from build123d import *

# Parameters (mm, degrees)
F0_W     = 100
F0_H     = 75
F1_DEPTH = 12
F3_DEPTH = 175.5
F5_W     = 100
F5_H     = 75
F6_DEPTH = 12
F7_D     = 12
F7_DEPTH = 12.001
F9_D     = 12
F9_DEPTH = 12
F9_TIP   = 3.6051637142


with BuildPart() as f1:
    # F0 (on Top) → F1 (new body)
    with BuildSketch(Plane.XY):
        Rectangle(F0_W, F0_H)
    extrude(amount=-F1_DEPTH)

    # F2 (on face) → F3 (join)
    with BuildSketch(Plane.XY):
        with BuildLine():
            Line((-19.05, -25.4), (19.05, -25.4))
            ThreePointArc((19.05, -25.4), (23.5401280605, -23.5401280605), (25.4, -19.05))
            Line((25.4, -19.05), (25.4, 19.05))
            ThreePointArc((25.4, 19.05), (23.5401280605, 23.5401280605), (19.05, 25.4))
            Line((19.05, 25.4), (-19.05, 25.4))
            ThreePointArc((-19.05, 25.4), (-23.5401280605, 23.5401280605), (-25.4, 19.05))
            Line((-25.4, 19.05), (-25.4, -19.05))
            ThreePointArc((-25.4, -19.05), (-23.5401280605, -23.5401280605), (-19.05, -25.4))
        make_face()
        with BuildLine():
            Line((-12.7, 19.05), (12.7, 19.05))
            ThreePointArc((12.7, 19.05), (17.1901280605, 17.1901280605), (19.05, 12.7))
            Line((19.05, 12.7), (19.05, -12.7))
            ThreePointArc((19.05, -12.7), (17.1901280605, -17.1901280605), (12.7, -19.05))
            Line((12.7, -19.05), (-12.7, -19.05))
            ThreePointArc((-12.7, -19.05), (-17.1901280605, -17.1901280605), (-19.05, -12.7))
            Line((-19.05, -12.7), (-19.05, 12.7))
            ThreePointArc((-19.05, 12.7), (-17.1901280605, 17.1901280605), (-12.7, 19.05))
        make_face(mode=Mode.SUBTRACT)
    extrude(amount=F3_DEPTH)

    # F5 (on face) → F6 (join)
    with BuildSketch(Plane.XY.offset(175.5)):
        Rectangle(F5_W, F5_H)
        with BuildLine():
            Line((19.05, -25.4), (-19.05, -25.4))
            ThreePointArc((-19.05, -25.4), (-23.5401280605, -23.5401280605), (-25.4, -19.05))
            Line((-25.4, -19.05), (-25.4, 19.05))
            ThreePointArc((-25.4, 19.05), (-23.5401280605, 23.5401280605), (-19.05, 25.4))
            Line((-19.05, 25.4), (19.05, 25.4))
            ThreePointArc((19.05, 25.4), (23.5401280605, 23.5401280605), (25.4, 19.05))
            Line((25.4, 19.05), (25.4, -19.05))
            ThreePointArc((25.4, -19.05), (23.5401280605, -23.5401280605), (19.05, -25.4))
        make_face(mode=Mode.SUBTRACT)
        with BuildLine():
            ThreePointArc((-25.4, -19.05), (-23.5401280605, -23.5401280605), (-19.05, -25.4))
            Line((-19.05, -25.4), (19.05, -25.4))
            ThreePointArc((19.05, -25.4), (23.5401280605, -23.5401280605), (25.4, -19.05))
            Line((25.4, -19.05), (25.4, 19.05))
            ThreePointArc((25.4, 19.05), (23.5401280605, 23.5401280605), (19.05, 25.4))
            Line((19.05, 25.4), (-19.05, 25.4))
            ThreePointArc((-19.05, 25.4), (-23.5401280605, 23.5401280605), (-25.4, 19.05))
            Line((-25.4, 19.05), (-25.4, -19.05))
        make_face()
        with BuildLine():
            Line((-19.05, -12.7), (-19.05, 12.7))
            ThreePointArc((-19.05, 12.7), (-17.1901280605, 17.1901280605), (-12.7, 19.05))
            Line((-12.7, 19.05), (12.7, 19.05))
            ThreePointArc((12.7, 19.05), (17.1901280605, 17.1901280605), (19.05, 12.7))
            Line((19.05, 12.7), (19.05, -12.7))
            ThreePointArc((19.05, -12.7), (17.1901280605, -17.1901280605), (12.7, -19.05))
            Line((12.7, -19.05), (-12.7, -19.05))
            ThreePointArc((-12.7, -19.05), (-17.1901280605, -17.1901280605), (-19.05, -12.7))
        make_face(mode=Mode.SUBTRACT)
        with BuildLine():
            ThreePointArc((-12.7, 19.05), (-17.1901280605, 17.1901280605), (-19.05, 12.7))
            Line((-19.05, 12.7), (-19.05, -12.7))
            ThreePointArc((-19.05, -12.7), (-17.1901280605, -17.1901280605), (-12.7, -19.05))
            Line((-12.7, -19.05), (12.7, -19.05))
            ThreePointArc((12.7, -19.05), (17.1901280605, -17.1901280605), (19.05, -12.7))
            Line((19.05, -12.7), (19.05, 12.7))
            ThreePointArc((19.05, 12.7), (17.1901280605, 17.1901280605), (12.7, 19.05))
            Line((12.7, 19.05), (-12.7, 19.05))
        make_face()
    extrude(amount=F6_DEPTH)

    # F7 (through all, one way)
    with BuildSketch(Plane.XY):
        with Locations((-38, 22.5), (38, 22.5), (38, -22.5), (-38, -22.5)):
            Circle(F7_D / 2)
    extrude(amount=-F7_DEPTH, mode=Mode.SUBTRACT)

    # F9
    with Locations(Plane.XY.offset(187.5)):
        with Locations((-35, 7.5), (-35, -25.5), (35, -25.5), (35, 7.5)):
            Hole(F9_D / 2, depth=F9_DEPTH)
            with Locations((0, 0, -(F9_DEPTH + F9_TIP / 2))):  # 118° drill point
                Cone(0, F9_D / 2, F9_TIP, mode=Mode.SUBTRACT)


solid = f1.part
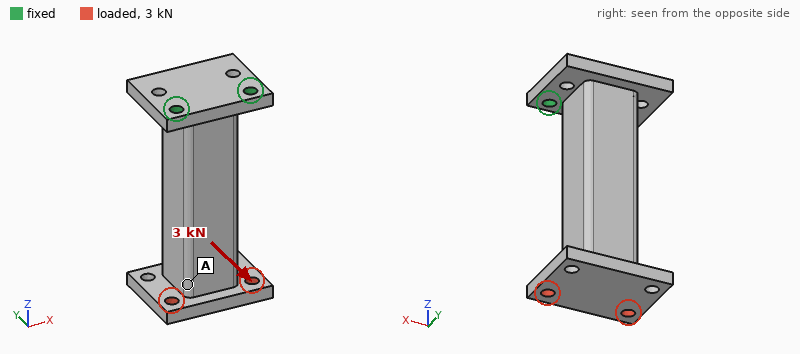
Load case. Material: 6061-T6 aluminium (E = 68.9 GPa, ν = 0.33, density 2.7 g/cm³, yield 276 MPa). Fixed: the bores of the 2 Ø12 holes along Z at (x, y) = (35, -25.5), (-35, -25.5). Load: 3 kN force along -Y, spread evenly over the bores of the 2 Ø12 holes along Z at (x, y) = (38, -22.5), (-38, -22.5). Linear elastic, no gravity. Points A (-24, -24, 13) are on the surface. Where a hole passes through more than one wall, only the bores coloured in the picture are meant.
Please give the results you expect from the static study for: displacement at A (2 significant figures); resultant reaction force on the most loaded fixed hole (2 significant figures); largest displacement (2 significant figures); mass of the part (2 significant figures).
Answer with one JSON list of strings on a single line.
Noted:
["1.7 mm", "1.8 kN", "2.1 mm", "990 g"]
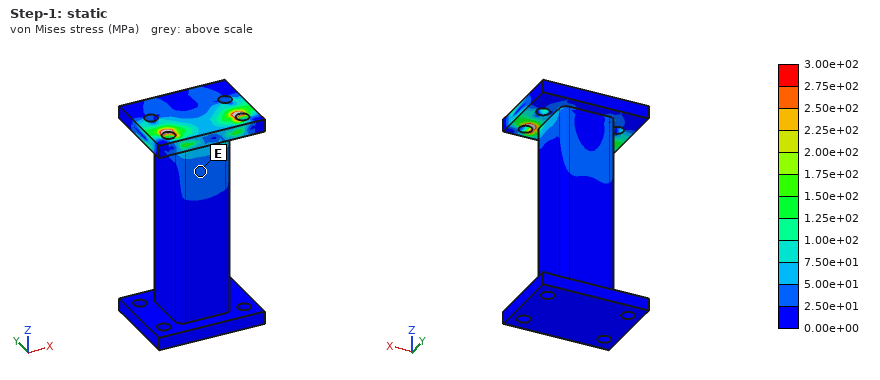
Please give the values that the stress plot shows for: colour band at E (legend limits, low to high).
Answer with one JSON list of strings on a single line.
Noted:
["2.50e+01 to 5.00e+01 MPa"]
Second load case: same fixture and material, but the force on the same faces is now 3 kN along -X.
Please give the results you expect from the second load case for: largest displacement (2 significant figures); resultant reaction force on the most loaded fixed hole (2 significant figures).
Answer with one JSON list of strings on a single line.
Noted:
["0.60 mm", "9.6 kN"]
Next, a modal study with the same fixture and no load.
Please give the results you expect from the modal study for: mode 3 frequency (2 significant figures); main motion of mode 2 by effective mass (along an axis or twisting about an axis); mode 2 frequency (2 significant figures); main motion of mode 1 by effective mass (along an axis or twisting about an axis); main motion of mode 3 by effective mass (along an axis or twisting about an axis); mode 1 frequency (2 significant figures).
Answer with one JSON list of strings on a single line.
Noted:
["2300 Hz", "along X", "620 Hz", "along Y", "twisting about Z", "310 Hz"]
